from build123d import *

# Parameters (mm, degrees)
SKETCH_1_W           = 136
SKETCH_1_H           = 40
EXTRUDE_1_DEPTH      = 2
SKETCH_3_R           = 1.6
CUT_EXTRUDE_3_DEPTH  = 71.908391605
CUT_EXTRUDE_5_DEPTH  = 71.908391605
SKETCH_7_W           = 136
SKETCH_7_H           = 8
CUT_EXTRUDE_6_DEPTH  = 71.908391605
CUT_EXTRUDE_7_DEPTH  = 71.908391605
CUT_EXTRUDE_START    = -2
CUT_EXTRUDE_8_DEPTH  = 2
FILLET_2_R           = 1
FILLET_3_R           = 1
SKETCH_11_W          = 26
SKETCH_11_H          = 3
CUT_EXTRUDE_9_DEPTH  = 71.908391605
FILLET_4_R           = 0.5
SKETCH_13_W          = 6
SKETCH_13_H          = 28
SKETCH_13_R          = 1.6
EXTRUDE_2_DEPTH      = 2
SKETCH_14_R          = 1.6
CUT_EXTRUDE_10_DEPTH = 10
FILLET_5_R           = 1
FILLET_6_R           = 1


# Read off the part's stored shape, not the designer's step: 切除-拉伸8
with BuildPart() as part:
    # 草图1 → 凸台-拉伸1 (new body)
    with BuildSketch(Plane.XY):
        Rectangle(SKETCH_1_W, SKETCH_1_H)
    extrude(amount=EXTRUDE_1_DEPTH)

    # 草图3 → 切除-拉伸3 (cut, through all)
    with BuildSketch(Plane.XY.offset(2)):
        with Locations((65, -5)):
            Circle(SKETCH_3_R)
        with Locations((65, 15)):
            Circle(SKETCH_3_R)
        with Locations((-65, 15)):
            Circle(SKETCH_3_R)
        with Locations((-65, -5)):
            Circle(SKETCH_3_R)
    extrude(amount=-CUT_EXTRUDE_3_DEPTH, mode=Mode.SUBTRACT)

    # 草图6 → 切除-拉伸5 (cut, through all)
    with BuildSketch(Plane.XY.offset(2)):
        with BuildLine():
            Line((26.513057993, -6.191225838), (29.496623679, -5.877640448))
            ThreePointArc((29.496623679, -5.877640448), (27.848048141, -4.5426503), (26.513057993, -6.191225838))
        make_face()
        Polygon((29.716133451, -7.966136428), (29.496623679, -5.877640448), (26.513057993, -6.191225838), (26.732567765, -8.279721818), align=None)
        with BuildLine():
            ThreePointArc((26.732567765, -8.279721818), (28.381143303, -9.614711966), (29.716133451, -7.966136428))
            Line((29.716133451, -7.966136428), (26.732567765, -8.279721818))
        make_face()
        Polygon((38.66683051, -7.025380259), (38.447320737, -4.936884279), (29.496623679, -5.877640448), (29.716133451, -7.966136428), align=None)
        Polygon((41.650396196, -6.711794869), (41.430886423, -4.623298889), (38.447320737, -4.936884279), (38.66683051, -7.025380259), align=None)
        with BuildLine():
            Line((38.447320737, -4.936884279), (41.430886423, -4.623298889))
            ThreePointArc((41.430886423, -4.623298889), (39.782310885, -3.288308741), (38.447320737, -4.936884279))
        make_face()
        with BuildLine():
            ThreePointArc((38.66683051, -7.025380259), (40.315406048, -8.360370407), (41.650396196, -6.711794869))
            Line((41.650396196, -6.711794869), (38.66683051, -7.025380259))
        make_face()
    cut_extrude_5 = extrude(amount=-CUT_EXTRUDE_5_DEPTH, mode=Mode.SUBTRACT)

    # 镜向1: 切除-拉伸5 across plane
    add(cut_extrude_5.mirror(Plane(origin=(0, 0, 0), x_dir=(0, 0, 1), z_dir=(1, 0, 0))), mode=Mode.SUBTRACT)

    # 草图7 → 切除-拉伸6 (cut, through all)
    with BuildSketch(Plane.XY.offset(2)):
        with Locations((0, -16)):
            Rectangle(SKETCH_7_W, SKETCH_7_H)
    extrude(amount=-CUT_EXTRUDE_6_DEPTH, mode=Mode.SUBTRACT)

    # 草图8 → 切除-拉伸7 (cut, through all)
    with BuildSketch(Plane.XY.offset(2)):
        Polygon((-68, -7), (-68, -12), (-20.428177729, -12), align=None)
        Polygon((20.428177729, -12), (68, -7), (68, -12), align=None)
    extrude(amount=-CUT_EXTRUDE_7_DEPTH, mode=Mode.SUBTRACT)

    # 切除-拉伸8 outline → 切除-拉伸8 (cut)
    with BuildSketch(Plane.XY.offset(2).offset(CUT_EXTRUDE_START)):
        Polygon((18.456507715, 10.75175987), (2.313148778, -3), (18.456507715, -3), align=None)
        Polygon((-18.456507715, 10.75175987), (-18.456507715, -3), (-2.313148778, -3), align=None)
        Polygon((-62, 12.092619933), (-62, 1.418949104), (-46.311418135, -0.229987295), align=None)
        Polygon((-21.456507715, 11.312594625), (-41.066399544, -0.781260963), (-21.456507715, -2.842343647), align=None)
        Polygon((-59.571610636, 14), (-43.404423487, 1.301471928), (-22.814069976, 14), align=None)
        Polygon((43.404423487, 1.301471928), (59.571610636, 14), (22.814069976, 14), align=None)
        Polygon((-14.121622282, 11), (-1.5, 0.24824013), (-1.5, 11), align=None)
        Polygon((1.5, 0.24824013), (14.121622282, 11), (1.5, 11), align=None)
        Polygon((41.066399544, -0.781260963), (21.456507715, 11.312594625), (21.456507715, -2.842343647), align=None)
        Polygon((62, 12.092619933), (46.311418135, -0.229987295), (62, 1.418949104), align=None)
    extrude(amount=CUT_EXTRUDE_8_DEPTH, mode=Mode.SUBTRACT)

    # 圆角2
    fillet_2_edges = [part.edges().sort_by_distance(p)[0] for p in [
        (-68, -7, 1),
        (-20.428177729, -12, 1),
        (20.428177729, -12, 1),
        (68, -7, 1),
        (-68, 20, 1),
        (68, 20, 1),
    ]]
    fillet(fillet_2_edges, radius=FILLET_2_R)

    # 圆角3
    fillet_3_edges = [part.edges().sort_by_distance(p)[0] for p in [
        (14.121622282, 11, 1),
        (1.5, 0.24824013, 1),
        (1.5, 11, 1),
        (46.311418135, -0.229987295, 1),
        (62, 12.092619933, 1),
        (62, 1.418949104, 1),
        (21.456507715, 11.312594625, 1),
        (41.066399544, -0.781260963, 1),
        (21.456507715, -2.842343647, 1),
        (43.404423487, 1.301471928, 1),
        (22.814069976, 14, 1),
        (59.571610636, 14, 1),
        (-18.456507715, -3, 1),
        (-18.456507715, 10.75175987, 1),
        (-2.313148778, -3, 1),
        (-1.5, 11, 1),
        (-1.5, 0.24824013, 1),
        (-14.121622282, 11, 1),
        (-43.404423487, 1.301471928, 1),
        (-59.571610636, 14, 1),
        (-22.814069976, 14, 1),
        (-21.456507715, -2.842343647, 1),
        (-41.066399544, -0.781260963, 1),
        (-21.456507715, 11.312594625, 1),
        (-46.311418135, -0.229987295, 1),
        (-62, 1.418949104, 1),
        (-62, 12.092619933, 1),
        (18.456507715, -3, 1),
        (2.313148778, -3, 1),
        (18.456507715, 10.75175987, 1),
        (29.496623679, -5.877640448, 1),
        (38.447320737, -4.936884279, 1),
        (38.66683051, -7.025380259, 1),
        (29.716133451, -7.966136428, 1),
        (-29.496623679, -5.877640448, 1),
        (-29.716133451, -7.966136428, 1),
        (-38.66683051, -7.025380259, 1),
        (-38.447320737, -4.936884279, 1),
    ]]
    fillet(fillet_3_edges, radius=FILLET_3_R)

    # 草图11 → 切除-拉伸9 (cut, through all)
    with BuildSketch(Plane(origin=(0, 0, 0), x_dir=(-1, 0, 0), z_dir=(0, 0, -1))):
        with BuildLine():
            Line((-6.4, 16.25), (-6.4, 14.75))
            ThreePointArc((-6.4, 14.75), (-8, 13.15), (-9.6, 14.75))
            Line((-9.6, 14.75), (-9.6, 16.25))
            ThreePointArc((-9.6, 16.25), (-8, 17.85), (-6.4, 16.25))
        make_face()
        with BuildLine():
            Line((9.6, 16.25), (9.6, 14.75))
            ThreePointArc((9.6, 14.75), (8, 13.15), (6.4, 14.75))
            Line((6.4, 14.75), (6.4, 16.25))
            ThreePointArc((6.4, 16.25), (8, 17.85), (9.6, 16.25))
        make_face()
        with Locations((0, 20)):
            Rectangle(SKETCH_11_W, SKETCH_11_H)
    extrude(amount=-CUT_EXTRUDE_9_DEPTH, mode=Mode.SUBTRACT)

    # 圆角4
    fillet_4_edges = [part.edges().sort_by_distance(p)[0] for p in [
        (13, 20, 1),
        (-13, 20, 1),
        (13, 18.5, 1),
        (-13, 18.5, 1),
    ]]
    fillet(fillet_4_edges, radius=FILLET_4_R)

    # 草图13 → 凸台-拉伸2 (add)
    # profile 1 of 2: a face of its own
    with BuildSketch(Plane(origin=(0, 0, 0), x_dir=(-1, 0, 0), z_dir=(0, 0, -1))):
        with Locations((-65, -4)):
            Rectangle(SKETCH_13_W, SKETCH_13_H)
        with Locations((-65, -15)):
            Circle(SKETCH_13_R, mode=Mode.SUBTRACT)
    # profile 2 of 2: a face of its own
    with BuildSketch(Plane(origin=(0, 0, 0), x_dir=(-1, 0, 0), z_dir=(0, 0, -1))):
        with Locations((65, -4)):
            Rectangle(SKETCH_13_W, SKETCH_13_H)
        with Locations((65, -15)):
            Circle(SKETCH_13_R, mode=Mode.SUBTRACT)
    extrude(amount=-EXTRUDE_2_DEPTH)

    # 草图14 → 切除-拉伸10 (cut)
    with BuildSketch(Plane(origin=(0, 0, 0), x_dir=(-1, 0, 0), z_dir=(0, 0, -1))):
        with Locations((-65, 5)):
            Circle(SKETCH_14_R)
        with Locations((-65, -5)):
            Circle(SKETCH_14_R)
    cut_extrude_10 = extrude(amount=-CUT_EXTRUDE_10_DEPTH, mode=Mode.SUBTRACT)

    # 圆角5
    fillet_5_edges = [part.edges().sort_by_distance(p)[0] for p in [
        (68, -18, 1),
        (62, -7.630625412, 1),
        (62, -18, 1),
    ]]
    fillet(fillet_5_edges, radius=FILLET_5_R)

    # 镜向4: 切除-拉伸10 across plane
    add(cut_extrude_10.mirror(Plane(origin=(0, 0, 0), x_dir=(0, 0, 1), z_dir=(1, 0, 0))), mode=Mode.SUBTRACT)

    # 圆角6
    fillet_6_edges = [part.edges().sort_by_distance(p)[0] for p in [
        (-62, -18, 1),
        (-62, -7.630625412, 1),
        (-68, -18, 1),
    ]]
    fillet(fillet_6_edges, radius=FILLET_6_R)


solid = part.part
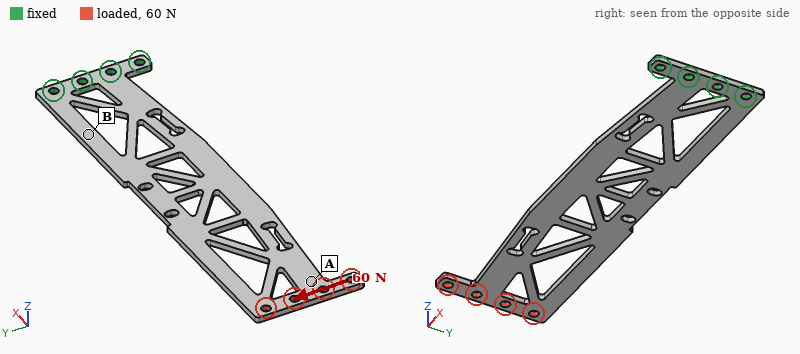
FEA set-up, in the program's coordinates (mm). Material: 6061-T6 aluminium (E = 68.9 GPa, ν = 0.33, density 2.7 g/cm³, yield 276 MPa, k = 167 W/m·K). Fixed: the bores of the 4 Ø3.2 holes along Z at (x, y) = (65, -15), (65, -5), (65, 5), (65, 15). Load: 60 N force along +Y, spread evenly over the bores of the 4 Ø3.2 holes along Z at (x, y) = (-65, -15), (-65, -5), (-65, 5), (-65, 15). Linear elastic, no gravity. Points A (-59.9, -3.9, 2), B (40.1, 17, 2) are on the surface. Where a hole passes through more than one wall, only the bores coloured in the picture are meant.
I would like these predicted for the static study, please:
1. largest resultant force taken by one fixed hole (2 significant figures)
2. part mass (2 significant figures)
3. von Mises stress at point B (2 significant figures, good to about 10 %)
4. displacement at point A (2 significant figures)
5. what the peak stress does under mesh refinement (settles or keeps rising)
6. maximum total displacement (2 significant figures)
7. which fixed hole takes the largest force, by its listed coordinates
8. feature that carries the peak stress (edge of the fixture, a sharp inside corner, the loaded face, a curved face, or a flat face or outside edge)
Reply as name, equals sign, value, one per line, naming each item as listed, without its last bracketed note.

largest resultant force taken by one fixed hole = 370 N
part mass = 15 g
von Mises stress at point B = 25 MPa
displacement at point A = 0.23 mm
what the peak stress does under mesh refinement = keeps rising
maximum total displacement = 0.26 mm
which fixed hole takes the largest force, by its listed coordinates = (65, 15)
feature that carries the peak stress = a sharp inside corner
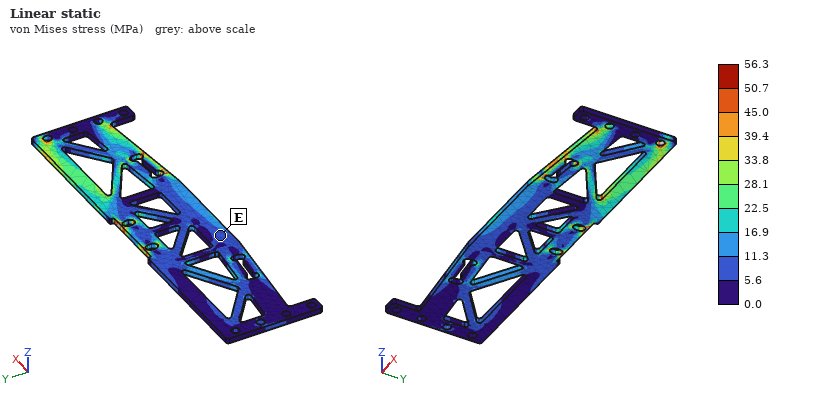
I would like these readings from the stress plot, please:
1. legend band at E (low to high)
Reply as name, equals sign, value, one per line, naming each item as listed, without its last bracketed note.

legend band at E = 5.6 to 11.3 MPa
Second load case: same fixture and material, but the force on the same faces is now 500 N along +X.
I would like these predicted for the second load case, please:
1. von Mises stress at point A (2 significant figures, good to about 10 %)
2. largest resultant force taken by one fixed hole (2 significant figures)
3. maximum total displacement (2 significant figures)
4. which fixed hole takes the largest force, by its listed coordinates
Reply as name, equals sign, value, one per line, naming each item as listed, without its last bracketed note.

von Mises stress at point A = 16 MPa
largest resultant force taken by one fixed hole = 330 N
maximum total displacement = 0.13 mm
which fixed hole takes the largest force, by its listed coordinates = (65, -5)
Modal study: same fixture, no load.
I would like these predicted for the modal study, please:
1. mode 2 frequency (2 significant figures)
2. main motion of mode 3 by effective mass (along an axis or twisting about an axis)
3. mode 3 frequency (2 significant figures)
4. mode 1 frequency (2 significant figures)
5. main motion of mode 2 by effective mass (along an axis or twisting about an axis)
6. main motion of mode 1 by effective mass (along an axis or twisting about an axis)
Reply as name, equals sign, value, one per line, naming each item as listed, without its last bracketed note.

mode 2 frequency = 510 Hz
main motion of mode 3 by effective mass = twisting about X
mode 3 frequency = 590 Hz
mode 1 frequency = 83 Hz
main motion of mode 2 by effective mass = along Z
main motion of mode 1 by effective mass = along Z
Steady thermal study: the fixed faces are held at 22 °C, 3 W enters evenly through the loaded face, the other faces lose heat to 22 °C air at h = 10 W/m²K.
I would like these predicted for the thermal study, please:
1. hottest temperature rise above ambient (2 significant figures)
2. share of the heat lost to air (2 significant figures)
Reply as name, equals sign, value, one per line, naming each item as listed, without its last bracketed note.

hottest temperature rise above ambient = 51 K
share of the heat lost to air = 50 %
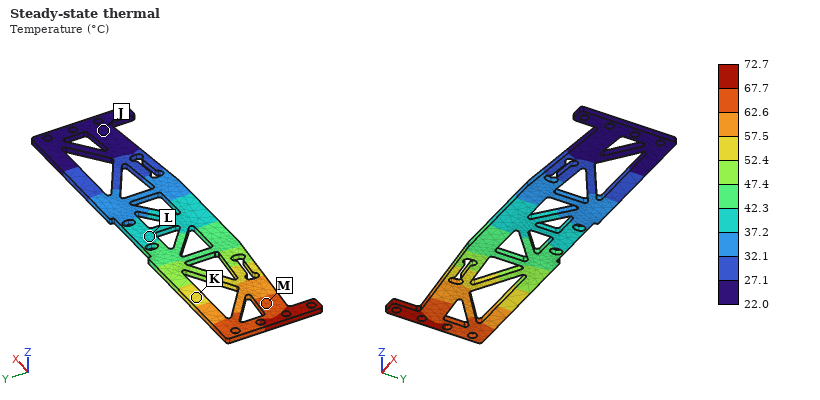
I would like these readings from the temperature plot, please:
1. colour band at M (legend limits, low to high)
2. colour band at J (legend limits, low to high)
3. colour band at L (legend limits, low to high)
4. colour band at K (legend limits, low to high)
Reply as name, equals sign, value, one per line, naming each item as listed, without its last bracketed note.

colour band at M = 62.6 to 67.7 °C
colour band at J = 22.0 to 27.1 °C
colour band at L = 37.2 to 42.3 °C
colour band at K = 52.4 to 57.5 °C
